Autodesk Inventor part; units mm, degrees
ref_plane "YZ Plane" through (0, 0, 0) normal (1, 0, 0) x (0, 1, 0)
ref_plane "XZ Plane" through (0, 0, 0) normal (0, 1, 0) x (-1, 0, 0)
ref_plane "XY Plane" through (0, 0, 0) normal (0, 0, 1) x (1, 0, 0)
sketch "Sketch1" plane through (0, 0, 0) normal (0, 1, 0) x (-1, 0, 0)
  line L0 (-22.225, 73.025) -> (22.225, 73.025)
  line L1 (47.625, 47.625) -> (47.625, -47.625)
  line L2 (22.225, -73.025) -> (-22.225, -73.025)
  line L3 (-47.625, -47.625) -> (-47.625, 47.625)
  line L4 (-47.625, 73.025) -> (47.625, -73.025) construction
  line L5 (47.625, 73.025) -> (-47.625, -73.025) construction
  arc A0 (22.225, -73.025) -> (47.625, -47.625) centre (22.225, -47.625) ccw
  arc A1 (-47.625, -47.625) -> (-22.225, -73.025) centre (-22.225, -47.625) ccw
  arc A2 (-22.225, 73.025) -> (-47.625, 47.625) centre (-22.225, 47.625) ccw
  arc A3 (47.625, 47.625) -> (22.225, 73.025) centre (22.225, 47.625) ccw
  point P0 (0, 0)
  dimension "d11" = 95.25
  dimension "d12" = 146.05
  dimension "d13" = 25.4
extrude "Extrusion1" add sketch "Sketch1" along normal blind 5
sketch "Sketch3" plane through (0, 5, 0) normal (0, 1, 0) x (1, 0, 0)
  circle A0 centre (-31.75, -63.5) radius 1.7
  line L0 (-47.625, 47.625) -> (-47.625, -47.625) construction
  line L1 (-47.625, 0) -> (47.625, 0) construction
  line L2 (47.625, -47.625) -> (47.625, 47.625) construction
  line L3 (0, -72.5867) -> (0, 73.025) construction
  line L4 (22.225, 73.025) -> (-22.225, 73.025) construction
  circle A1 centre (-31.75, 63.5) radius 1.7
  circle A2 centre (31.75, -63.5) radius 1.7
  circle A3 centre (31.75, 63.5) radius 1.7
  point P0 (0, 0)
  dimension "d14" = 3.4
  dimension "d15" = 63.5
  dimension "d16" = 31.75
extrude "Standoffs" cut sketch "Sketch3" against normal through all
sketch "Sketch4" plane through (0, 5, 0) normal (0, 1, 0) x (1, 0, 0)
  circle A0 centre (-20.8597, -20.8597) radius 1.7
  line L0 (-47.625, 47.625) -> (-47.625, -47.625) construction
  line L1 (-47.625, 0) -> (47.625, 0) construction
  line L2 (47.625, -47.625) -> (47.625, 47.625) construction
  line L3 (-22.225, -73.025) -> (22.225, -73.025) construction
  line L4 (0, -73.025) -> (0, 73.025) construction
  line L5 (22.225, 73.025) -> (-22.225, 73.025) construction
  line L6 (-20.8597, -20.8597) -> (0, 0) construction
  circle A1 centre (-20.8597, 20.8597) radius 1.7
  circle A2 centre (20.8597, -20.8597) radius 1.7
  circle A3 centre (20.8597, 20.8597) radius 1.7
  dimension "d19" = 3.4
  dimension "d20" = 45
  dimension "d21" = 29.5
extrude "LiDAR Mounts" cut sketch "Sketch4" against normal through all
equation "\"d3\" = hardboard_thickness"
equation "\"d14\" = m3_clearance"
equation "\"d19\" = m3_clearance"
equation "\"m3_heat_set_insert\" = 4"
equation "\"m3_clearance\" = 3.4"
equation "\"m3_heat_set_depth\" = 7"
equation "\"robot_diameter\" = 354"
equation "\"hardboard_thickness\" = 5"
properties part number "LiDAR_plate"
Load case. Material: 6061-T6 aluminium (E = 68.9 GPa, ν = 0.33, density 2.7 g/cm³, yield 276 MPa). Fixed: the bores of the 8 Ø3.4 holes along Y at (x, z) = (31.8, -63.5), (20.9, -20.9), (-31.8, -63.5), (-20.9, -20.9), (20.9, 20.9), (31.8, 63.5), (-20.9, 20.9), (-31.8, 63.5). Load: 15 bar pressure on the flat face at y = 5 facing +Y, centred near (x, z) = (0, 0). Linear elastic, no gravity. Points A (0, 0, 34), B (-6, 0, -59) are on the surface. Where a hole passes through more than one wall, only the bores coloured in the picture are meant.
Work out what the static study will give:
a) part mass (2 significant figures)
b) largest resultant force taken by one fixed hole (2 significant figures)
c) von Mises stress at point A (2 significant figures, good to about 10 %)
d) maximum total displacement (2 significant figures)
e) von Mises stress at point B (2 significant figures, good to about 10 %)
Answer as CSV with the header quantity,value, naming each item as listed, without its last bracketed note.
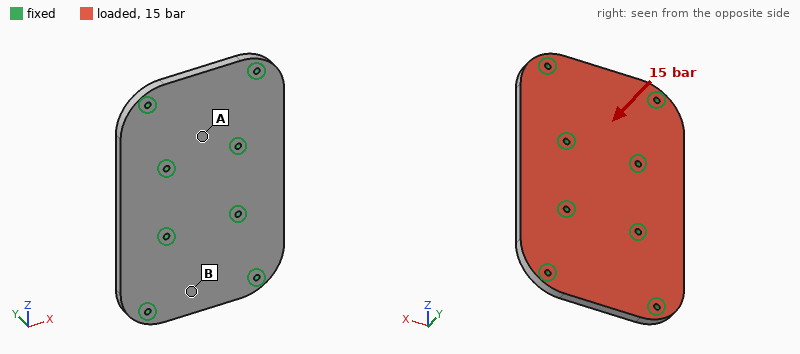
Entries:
quantity,value
part mass,180 g
largest resultant force taken by one fixed hole,3.1 kN
von Mises stress at point A,23 MPa
maximum total displacement,0.16 mm
von Mises stress at point B,42 MPa
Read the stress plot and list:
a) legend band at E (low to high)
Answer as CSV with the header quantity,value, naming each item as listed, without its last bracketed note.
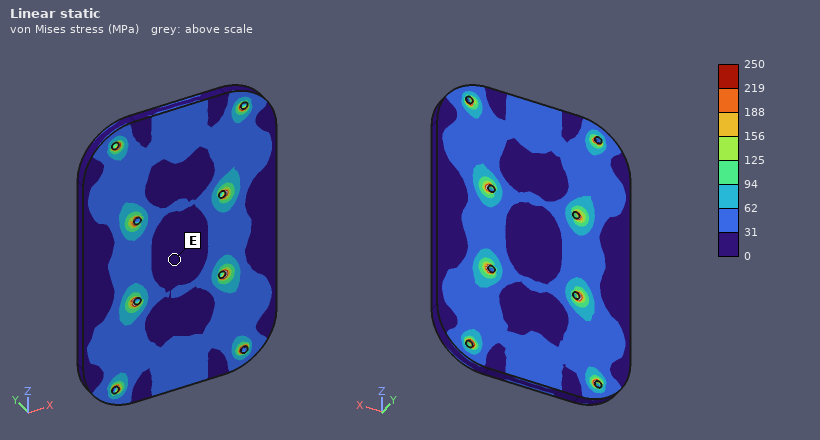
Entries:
quantity,value
legend band at E,0 to 31 MPa
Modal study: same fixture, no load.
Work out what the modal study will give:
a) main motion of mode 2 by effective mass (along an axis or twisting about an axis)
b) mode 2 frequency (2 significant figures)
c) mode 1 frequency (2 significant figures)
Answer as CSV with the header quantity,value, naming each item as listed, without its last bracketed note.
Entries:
quantity,value
main motion of mode 2 by effective mass,twisting about Z
mode 2 frequency,5200 Hz
mode 1 frequency,4900 Hz
